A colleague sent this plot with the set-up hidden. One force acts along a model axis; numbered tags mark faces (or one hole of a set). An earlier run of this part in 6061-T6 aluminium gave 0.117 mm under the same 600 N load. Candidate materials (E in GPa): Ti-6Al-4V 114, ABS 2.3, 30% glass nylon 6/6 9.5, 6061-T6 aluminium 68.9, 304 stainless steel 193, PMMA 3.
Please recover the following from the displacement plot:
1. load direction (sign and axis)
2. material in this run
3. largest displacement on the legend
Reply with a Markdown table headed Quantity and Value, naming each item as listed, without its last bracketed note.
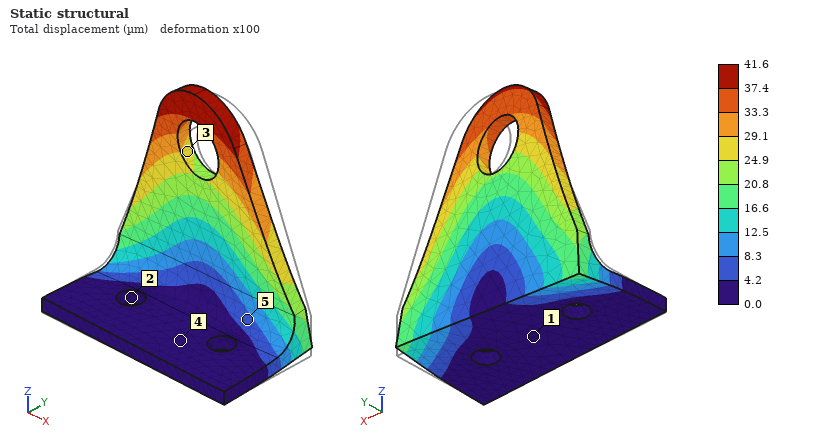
| Quantity | Value |
|---|---|
| load direction | -X |
| material in this run | 304 stainless steel |
| largest displacement on the legend | 41.6 µm |
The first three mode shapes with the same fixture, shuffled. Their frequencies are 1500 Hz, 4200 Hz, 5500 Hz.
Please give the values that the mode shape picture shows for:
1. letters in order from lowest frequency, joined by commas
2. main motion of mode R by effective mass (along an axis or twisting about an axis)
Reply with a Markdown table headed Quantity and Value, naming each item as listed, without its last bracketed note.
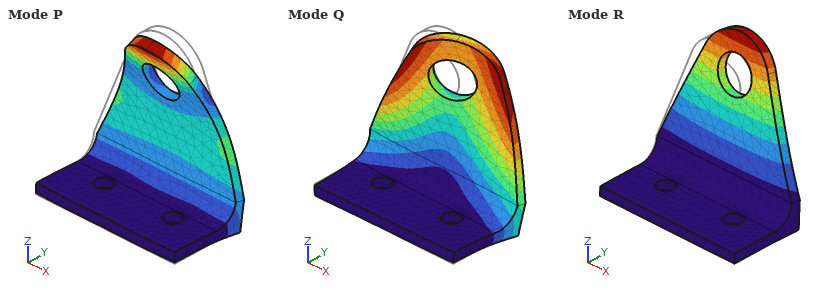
| Quantity | Value |
|---|---|
| letters in order from lowest frequency, joined by commas | R, Q, P |
| main motion of mode R by effective mass | along Y |
